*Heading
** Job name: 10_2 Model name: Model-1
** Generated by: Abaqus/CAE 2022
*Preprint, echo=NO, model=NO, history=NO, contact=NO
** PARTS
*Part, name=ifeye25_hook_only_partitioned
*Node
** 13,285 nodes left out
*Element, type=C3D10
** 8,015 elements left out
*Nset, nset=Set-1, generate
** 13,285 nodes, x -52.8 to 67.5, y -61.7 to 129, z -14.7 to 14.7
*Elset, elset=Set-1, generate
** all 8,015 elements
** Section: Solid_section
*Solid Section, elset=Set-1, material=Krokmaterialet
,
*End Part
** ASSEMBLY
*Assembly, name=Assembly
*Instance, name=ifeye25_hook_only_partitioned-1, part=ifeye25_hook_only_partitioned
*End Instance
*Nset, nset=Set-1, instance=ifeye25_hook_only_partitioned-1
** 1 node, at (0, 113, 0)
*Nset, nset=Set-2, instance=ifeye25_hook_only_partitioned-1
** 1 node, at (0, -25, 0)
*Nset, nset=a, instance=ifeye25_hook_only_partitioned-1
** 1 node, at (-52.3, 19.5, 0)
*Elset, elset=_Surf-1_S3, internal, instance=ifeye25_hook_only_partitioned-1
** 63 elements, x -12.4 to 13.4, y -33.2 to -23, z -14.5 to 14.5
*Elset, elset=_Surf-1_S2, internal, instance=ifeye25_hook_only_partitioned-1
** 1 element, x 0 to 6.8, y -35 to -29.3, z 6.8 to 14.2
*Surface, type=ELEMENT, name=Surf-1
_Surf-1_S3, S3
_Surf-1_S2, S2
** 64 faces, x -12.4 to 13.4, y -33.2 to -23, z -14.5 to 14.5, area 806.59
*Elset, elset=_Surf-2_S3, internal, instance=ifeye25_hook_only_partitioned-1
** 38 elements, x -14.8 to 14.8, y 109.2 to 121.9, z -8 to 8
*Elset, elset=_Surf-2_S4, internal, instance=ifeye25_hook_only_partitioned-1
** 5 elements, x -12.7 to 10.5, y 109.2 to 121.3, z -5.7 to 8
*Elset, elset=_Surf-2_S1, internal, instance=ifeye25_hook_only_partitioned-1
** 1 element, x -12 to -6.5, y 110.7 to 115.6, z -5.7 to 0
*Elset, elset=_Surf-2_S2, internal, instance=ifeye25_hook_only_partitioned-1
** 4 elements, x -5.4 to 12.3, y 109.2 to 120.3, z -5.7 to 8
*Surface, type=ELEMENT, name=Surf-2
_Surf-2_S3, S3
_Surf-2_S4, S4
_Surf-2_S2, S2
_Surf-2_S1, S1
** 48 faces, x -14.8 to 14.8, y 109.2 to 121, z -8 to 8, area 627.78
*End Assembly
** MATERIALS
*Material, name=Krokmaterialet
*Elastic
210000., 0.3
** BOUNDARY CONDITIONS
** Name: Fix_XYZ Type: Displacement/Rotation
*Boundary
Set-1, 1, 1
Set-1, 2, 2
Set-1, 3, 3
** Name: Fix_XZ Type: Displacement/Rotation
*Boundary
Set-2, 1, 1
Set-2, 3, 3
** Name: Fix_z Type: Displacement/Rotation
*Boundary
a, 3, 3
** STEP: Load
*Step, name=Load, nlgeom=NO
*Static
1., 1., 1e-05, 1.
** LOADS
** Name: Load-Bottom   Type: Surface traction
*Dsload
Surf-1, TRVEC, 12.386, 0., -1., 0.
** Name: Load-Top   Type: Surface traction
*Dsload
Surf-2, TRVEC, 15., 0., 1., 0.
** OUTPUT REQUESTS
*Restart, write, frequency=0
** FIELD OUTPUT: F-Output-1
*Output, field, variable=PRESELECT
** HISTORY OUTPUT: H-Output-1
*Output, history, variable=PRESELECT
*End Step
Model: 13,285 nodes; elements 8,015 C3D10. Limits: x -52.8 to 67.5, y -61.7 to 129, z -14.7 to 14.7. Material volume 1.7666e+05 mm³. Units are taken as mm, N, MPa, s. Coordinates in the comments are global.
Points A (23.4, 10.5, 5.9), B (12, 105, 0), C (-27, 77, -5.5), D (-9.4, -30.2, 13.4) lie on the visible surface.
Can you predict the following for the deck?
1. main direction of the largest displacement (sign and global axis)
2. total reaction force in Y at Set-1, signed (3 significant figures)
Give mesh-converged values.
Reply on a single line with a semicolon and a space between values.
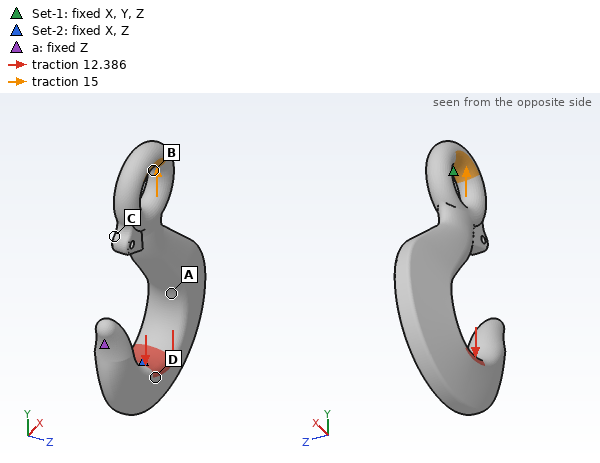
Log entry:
-Y; 574 N
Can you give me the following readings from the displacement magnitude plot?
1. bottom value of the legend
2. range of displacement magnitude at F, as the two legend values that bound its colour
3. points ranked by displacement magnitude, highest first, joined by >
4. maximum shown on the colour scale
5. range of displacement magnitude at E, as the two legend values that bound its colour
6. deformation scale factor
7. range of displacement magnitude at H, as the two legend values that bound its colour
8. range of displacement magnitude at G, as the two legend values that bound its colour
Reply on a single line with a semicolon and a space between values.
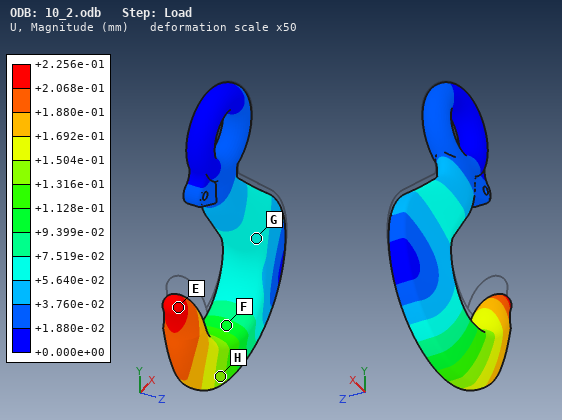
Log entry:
+0.000e+00 mm; +9.399e-02 to +1.128e-01 mm; E > H > F > G; +2.256e-01 mm; +2.068e-01 to +2.256e-01 mm; 50; +1.316e-01 to +1.504e-01 mm; +5.640e-02 to +7.519e-02 mm
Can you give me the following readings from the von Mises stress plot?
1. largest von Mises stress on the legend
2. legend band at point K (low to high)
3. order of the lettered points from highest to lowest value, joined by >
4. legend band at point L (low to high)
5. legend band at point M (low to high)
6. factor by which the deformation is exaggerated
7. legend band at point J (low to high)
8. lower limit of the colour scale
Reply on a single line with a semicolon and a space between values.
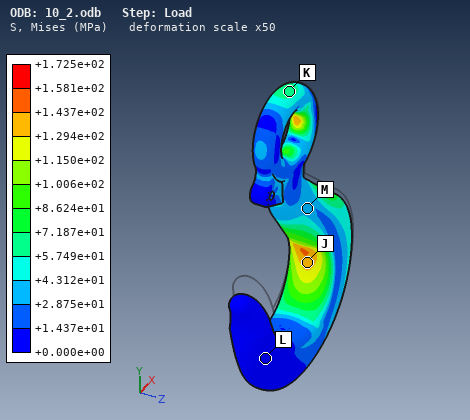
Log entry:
+1.725e+02 MPa; +5.749e+01 to +7.187e+01 MPa; J > K > M > L; +0.000e+00 to +1.437e+01 MPa; +2.875e+01 to +4.312e+01 MPa; 50; +1.294e+02 to +1.437e+02 MPa; +0.000e+00 MPa
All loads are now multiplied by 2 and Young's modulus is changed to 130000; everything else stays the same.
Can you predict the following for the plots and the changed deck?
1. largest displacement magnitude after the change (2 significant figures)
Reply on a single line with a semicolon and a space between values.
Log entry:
0.73 mm
